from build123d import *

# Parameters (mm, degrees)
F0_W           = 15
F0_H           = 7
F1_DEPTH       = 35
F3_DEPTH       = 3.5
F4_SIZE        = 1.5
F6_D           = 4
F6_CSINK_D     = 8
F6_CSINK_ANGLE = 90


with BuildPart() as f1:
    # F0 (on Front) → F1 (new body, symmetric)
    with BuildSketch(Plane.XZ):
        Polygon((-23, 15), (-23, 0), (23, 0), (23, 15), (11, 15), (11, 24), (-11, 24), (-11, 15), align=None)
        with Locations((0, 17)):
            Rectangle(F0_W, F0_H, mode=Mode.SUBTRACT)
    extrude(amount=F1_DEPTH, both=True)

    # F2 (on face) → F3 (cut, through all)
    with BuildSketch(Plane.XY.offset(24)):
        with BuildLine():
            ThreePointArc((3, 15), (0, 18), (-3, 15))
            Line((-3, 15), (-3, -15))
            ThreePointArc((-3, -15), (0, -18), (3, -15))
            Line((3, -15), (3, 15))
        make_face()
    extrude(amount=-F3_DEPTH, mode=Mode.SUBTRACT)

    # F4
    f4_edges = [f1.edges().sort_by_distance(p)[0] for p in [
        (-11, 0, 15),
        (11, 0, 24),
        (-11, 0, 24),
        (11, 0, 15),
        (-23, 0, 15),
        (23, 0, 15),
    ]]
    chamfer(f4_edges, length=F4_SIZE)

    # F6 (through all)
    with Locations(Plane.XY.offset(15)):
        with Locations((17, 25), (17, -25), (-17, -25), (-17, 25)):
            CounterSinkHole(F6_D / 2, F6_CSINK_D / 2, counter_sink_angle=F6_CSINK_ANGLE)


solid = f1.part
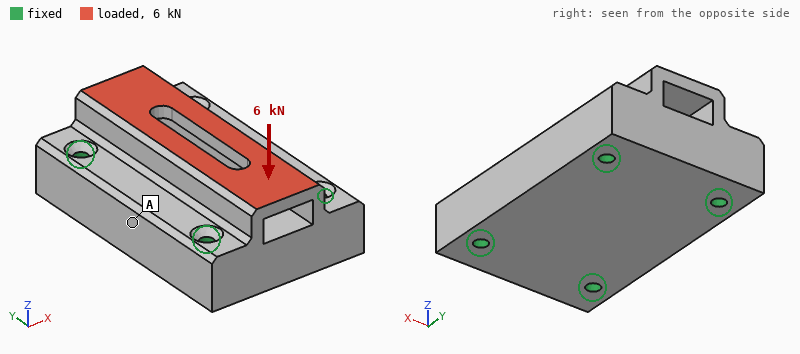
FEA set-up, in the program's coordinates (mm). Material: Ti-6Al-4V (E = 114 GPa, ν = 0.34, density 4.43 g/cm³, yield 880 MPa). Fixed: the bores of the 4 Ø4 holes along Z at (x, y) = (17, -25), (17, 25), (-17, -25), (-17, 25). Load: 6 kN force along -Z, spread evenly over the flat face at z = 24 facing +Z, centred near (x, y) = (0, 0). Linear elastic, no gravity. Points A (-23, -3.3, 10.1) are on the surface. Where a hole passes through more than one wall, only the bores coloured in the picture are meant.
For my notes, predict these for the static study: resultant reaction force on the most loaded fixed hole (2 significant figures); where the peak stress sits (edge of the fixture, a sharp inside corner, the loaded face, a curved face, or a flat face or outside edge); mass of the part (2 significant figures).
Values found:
1.6 kN
the loaded face
230 g
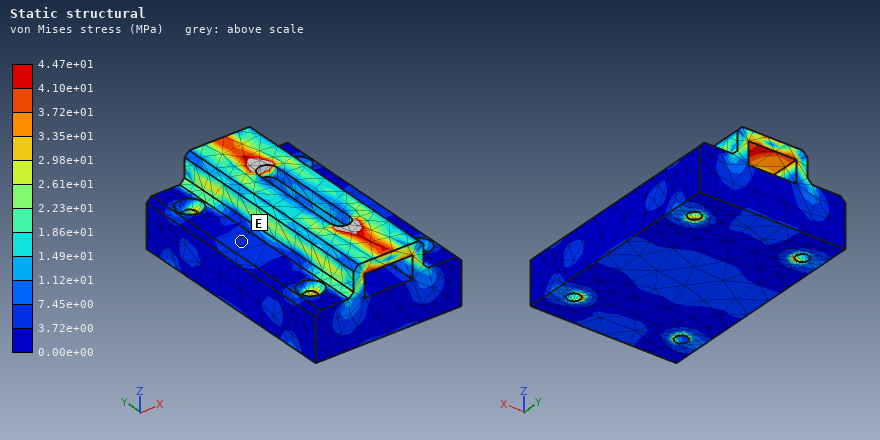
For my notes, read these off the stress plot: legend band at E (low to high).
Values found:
3.72e+00 to 7.45e+00 MPa
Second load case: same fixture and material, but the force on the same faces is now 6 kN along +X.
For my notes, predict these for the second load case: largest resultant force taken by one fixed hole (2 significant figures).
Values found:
2.0 kN
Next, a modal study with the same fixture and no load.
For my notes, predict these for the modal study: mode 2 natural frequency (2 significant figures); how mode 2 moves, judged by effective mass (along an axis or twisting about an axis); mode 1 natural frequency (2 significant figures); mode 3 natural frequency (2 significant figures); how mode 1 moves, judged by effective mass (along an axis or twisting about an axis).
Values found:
21 kHz
along X
17 kHz
24 kHz
along Z
